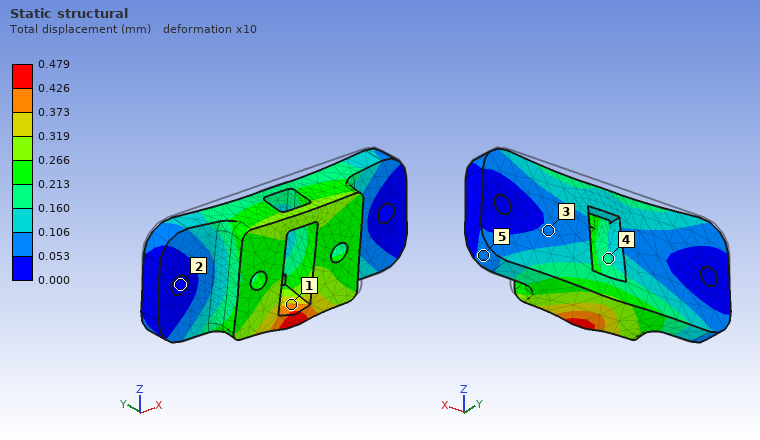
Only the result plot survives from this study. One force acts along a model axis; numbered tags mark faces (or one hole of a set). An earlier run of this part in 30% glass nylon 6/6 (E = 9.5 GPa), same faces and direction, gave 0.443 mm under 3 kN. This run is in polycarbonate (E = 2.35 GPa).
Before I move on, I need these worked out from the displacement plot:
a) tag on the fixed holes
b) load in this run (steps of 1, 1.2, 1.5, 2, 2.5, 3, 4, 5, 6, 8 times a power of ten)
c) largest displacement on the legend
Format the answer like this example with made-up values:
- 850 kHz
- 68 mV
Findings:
- 2
- 800 N
- 0.479 mm
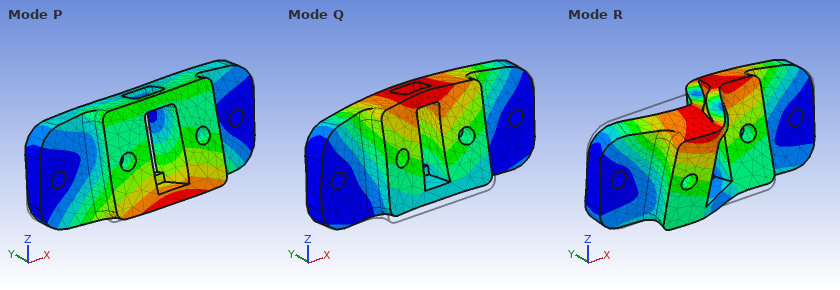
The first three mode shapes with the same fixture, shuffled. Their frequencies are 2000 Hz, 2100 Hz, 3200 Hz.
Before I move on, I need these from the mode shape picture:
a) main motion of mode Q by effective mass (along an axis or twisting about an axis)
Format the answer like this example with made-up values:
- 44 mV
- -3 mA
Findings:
- along Y
